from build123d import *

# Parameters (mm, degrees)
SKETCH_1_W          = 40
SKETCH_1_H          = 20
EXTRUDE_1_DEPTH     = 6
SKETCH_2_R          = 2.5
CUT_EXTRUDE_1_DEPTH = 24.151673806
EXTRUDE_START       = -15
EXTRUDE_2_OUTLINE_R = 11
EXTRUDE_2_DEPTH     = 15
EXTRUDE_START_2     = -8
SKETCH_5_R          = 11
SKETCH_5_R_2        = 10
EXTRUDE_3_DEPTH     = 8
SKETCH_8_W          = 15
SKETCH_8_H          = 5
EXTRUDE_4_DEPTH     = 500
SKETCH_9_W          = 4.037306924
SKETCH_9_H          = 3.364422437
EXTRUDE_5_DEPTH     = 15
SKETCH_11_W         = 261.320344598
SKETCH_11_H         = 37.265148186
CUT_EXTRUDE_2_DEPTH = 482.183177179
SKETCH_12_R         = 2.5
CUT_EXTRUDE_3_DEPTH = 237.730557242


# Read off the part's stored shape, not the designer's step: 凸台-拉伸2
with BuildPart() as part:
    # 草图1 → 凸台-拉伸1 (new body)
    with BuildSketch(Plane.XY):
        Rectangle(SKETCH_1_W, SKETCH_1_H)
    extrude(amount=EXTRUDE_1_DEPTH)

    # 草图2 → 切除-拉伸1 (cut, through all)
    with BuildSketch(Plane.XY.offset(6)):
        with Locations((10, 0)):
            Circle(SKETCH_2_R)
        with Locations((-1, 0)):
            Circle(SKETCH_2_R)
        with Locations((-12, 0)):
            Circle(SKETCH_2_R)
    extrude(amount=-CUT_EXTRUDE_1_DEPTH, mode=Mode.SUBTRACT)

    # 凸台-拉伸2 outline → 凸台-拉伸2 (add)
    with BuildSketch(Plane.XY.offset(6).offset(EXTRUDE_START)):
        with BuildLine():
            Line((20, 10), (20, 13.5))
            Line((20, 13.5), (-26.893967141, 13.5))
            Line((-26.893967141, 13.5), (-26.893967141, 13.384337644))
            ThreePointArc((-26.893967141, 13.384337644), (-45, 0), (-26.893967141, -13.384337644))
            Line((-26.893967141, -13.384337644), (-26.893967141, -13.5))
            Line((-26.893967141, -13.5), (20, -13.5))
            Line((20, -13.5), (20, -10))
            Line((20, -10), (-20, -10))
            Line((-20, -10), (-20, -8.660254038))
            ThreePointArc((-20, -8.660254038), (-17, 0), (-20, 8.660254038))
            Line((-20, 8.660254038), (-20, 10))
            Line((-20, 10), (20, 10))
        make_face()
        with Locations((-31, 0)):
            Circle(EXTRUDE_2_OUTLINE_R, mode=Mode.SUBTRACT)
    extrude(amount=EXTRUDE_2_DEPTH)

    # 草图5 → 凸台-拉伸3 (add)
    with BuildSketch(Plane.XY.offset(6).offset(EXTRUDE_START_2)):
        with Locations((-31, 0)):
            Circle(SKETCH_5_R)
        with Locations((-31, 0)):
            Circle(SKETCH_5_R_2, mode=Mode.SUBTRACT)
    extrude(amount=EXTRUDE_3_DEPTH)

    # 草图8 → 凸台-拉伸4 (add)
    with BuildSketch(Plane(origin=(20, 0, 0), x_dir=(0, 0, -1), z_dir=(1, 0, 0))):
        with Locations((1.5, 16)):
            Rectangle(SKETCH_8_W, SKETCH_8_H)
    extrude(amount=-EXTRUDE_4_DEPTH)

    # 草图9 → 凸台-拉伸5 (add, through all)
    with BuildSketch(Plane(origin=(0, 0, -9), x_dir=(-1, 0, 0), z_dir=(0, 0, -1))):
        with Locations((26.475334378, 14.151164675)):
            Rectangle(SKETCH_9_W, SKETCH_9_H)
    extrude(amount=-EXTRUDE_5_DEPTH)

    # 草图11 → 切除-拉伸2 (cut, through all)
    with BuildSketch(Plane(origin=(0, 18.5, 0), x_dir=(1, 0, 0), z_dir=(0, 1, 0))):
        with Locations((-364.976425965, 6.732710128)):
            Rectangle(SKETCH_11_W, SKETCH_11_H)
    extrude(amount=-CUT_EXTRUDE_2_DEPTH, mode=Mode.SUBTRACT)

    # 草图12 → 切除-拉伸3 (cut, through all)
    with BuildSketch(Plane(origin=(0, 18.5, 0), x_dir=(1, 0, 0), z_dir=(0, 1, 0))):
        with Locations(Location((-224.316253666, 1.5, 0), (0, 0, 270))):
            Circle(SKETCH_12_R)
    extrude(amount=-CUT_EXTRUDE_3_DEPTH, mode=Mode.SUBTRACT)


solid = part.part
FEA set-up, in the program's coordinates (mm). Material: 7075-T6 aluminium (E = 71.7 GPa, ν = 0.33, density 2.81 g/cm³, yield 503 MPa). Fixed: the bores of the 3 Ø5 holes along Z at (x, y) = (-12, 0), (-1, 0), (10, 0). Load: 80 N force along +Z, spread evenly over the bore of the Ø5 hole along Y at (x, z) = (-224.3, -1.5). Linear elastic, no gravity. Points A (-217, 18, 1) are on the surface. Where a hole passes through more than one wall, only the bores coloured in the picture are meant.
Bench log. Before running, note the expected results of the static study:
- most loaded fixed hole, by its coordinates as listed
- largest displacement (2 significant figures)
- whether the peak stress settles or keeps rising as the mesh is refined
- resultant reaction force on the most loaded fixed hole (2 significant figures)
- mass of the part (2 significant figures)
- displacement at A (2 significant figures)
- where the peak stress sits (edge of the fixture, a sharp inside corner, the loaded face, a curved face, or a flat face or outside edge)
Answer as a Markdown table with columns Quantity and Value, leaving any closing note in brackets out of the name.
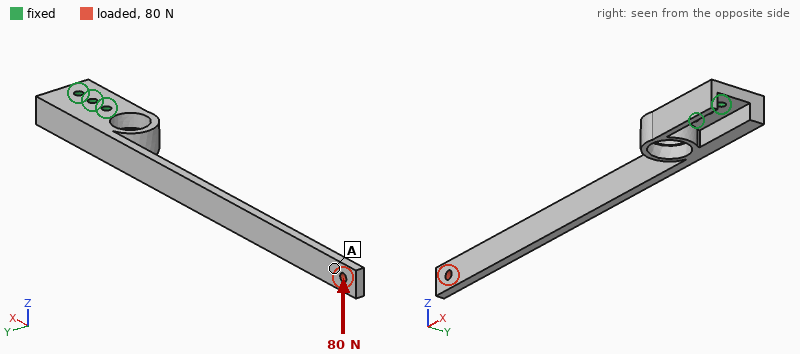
| Quantity | Value |
|---|---|
| most loaded fixed hole, by its coordinates as listed | (-12, 0) |
| largest displacement | 2.5 mm |
| whether the peak stress settles or keeps rising as the mesh is refined | keeps rising |
| resultant reaction force on the most loaded fixed hole | 720 N |
| mass of the part | 89 g |
| displacement at A | 2.2 mm |
| where the peak stress sits | edge of the fixture |
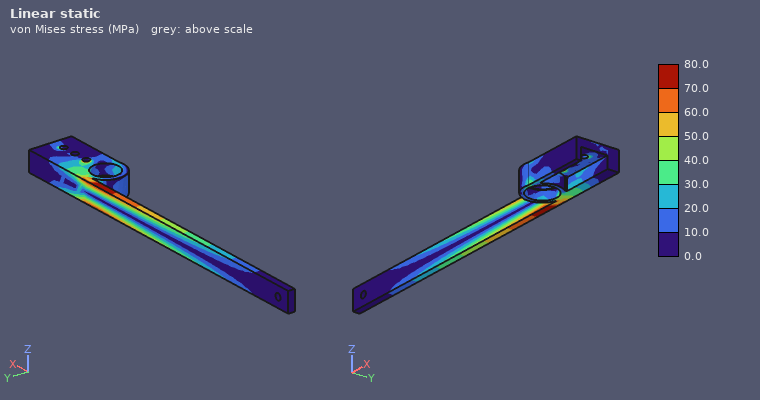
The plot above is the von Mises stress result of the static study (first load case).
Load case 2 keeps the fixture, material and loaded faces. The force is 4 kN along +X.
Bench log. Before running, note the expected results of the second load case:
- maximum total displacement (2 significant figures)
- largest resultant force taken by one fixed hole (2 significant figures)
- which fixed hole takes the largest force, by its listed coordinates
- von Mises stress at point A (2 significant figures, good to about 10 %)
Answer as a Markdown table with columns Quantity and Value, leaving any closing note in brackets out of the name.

| Quantity | Value |
|---|---|
| maximum total displacement | 0.58 mm |
| largest resultant force taken by one fixed hole | 3.0 kN |
| which fixed hole takes the largest force, by its listed coordinates | (-12, 0) |
| von Mises stress at point A | 57 MPa |
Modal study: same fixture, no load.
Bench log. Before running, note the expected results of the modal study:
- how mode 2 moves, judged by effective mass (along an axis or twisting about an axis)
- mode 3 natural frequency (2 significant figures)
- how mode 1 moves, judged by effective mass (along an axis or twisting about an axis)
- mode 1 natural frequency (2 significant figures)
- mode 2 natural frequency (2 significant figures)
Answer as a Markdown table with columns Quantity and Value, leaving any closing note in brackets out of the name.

| Quantity | Value |
|---|---|
| how mode 2 moves, judged by effective mass | along Z |
| mode 3 natural frequency | 620 Hz |
| how mode 1 moves, judged by effective mass | along Y |
| mode 1 natural frequency | 100 Hz |
| mode 2 natural frequency | 260 Hz |
